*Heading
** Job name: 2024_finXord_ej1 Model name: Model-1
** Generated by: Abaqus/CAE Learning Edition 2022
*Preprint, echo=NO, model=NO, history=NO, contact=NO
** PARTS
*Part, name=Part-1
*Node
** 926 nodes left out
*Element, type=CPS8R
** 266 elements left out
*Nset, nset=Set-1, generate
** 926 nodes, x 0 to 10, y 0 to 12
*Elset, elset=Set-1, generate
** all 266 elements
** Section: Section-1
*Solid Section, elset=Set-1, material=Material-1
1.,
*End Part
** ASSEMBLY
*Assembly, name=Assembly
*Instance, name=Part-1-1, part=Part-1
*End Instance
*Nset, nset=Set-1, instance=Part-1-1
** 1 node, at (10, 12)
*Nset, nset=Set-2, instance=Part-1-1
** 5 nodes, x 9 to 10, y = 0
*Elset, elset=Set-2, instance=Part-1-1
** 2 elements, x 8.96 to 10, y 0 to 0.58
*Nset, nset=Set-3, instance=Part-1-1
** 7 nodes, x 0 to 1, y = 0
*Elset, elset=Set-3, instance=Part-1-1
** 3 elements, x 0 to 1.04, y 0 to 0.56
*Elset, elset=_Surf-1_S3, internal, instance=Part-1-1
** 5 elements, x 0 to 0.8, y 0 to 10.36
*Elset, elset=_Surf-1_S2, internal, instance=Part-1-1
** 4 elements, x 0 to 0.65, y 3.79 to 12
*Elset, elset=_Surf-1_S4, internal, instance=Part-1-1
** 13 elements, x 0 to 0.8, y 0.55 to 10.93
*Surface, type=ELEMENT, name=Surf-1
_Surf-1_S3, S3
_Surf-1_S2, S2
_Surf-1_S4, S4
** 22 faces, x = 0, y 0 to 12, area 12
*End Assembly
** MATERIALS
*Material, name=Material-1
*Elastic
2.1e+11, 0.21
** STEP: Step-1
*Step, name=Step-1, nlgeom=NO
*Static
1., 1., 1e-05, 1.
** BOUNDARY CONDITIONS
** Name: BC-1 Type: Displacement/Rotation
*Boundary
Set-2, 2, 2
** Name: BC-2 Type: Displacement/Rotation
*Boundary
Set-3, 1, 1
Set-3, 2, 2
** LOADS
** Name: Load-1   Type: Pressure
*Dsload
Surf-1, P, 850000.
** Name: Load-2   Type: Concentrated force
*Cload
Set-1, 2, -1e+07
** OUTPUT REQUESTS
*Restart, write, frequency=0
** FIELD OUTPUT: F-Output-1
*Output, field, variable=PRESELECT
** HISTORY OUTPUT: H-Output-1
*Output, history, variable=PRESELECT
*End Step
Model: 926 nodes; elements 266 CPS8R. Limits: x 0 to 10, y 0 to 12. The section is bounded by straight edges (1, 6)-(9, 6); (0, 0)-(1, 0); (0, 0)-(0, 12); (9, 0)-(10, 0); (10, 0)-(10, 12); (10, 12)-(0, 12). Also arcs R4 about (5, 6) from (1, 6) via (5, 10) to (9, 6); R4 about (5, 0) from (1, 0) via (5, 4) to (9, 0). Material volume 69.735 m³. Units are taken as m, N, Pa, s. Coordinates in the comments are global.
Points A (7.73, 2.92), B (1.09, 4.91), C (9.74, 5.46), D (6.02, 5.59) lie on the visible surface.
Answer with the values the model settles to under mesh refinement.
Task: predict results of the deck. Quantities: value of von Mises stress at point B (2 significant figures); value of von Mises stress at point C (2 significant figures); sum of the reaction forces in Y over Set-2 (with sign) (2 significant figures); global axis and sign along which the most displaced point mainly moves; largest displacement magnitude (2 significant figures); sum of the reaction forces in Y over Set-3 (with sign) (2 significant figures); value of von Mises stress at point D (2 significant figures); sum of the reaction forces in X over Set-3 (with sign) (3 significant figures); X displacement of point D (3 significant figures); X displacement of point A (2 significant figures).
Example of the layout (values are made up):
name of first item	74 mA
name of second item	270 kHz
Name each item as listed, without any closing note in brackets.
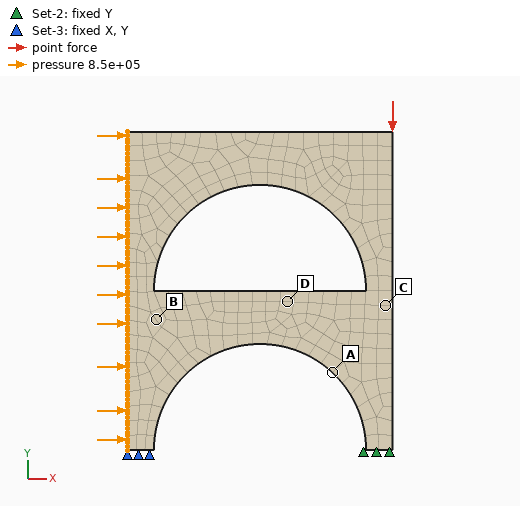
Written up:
value of von Mises stress at point B	6.4e+06 Pa
value of von Mises stress at point C	1.8e+07 Pa
sum of the reaction forces in Y over Set-2 (with sign)	1.6e+07 N
global axis and sign along which the most displaced point mainly moves	+X
largest displacement magnitude	0.0031 m
sum of the reaction forces in Y over Set-3 (with sign)	-6.3e+06 N
value of von Mises stress at point D	6.1e+06 Pa
sum of the reaction forces in X over Set-3 (with sign)	-1.02e+07 N
X displacement of point D	0.00175 m
X displacement of point A	0.0020 m
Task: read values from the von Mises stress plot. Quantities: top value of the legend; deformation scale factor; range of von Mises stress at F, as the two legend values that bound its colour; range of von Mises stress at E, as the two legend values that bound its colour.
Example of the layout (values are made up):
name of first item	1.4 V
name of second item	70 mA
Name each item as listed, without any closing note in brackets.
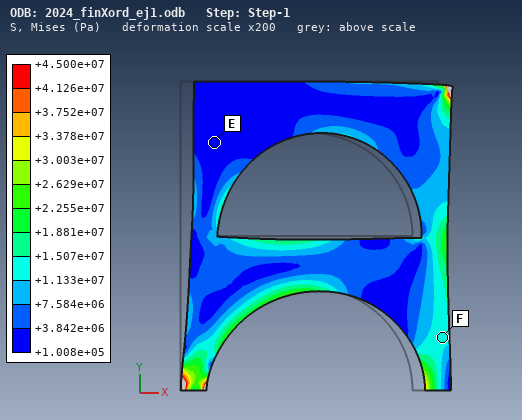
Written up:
top value of the legend	+4.500e+07 Pa
deformation scale factor	200
range of von Mises stress at F, as the two legend values that bound its colour	+1.133e+07 to +1.507e+07 Pa
range of von Mises stress at E, as the two legend values that bound its colour	+1.008e+05 to +3.842e+06 Pa
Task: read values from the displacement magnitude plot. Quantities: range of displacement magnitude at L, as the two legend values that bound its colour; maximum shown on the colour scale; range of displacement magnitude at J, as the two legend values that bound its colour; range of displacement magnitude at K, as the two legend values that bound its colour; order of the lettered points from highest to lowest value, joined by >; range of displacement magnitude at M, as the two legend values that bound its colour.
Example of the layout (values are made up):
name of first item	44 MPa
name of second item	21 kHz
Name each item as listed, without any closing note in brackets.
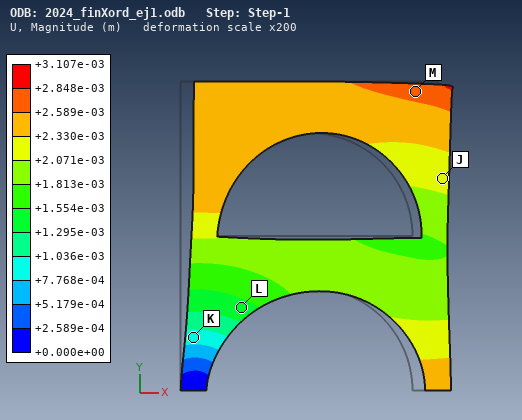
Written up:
range of displacement magnitude at L, as the two legend values that bound its colour	+1.295e-03 to +1.554e-03 m
maximum shown on the colour scale	+3.107e-03 m
range of displacement magnitude at J, as the two legend values that bound its colour	+2.071e-03 to +2.330e-03 m
range of displacement magnitude at K, as the two legend values that bound its colour	+7.768e-04 to +1.036e-03 m
order of the lettered points from highest to lowest value, joined by >	M > J > L > K
range of displacement magnitude at M, as the two legend values that bound its colour	+2.589e-03 to +2.848e-03 m
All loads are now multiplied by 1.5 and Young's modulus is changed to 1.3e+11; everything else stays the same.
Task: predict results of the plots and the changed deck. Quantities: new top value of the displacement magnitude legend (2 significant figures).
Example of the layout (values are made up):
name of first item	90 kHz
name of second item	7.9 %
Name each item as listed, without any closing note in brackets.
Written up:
new top value of the displacement magnitude legend	0.0075 m
